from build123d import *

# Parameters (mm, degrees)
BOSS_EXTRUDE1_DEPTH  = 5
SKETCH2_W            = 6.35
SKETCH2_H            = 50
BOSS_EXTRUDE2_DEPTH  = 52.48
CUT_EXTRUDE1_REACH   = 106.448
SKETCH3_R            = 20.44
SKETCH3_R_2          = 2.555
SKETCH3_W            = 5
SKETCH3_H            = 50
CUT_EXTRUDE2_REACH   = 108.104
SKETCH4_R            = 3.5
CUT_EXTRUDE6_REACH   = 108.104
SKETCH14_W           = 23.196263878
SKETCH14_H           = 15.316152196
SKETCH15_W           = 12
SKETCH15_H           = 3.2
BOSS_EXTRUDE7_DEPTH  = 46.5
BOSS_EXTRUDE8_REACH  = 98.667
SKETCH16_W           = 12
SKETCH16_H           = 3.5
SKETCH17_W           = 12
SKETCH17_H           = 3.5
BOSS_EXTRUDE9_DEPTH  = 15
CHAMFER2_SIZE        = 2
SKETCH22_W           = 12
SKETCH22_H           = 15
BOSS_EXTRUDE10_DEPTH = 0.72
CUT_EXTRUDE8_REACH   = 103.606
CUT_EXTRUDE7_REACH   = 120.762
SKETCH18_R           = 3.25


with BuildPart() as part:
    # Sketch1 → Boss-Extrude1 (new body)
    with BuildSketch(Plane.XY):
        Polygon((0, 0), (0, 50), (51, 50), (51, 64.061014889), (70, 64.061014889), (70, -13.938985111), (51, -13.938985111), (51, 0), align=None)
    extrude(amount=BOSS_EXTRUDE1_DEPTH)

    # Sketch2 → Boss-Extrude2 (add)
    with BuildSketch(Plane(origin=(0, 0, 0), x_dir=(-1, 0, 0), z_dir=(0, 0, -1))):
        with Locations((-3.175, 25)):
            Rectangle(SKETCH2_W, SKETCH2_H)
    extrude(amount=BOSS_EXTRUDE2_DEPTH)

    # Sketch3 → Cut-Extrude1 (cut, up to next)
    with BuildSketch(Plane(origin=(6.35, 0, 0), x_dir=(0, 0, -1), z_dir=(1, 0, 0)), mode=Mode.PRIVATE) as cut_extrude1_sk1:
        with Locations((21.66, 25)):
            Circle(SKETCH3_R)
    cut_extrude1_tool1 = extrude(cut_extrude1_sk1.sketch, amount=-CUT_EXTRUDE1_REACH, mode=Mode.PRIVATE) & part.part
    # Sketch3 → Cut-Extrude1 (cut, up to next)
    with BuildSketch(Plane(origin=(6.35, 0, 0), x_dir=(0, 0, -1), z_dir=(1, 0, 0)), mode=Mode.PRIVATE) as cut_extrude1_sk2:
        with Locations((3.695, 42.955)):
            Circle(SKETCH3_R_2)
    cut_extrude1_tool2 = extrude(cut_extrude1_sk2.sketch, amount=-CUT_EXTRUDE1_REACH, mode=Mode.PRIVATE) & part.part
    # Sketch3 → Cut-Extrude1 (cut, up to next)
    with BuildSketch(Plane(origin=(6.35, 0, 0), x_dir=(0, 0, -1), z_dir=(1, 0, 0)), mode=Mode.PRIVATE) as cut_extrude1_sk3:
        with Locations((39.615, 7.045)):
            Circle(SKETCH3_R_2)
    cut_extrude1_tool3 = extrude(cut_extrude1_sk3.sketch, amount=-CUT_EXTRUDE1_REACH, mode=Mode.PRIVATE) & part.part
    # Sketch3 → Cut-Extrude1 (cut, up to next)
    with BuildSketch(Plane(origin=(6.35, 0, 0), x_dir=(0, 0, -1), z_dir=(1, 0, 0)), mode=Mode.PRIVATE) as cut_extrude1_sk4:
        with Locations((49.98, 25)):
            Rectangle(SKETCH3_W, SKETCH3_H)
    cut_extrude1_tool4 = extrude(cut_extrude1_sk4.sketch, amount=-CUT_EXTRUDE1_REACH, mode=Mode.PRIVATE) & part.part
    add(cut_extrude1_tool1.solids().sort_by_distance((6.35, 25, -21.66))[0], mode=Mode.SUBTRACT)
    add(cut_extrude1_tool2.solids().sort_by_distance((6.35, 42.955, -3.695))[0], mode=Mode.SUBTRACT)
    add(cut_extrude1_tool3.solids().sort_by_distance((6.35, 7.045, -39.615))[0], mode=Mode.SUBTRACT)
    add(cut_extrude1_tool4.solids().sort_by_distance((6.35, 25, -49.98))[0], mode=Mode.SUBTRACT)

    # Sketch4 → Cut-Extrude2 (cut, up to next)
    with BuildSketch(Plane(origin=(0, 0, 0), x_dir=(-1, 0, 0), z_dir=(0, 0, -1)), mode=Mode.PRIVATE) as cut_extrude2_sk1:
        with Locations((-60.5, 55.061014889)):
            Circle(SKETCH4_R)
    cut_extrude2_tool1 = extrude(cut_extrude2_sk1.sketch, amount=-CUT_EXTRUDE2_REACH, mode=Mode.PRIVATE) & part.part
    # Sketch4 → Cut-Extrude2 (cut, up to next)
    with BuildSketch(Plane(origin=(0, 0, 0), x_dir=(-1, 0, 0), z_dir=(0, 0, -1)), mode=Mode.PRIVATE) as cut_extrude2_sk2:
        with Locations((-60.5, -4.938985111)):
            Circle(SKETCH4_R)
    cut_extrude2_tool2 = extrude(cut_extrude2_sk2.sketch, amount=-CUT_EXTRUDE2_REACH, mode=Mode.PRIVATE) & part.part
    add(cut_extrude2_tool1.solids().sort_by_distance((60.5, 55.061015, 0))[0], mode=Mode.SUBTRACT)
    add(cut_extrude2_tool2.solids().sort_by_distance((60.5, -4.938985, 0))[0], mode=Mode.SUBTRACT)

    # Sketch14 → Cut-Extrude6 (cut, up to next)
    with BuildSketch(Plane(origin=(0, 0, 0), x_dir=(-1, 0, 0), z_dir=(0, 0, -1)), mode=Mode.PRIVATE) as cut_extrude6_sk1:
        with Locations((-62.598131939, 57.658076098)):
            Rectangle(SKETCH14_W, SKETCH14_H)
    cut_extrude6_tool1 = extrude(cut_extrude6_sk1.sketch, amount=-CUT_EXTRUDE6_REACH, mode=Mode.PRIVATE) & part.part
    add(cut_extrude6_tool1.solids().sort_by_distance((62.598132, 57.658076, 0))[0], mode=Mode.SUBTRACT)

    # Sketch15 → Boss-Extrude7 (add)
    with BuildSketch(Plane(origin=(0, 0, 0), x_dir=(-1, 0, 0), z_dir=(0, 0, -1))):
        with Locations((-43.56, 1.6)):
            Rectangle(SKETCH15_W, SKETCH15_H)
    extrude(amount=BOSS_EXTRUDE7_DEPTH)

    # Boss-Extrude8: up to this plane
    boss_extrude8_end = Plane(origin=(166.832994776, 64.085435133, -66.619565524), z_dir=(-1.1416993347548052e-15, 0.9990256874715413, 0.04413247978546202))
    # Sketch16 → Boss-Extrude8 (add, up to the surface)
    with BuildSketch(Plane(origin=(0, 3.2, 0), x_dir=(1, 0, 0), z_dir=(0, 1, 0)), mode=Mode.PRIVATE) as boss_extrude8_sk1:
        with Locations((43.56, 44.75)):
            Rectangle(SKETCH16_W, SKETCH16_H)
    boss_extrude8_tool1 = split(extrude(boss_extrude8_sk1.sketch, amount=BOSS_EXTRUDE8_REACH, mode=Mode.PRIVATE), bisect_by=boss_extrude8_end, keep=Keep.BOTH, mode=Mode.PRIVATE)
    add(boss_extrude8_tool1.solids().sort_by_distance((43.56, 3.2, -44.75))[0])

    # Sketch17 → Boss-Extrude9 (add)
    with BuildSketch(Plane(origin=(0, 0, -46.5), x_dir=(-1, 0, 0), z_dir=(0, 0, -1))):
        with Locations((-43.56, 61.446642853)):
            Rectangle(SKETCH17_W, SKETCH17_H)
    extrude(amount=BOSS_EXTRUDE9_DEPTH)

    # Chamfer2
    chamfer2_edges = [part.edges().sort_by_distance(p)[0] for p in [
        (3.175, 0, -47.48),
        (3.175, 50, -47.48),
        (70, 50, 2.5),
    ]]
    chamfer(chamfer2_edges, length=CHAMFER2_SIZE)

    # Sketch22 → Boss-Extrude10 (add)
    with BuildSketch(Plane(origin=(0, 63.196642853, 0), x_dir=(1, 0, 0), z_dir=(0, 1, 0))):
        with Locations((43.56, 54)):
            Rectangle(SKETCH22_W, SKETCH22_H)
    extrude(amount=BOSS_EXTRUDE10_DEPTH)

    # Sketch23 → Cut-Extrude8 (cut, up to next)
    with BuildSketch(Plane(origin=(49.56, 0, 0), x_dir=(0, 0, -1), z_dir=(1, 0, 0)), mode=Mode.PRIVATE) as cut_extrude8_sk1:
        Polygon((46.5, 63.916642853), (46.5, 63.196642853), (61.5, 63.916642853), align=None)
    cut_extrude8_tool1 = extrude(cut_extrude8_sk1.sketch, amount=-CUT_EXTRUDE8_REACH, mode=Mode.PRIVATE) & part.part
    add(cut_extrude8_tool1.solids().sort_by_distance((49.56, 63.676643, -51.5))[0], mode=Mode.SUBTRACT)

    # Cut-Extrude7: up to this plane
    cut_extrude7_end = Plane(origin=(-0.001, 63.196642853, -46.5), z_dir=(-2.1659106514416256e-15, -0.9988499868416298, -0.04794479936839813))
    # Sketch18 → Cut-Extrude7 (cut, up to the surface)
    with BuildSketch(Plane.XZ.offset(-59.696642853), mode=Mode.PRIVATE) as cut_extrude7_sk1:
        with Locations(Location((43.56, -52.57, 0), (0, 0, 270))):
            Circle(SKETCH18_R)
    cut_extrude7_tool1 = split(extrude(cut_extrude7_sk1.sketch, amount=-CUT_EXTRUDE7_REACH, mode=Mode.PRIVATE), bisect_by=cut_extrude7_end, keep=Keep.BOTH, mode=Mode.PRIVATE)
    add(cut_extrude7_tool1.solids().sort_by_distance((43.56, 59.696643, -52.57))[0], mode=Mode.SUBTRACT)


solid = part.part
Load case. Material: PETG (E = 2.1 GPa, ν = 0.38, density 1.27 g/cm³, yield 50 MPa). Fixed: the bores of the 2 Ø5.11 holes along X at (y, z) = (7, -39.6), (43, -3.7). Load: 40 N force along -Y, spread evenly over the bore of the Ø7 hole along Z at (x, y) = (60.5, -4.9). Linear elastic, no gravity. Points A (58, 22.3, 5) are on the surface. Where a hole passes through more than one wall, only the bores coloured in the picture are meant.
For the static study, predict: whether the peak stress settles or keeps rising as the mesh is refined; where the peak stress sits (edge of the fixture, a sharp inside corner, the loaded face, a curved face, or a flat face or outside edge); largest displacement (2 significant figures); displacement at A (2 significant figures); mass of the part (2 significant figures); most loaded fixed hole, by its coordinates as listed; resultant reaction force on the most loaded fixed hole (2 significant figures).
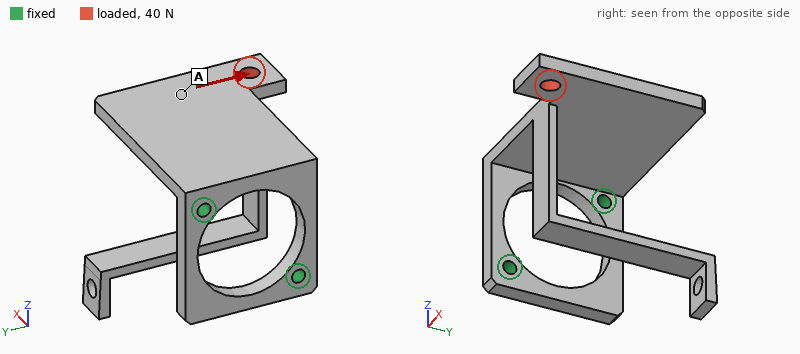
keeps rising
edge of the fixture
1.2 mm
0.78 mm
38 g
(43, -3.7)
42 N
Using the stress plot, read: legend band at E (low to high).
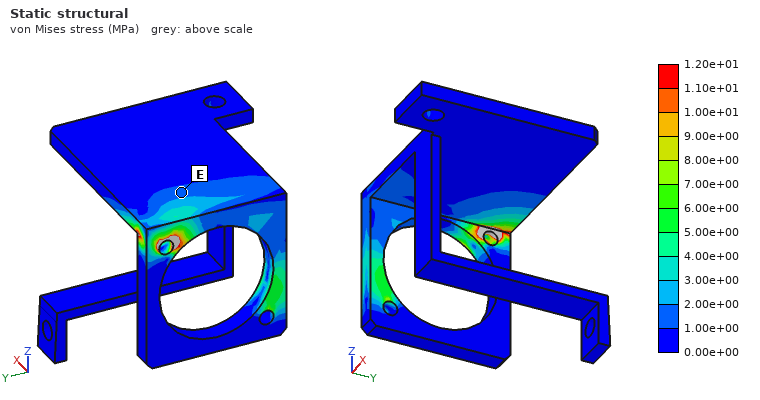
1.00e+00 to 2.00e+00 MPa
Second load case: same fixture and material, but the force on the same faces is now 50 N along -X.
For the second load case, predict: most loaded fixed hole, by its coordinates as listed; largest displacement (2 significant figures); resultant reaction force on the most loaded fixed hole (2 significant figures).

(43, -3.7)
1.3 mm
37 N
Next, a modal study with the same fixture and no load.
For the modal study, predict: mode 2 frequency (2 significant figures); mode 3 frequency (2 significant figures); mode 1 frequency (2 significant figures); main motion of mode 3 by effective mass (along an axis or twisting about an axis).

77 Hz
140 Hz
57 Hz
along Z
